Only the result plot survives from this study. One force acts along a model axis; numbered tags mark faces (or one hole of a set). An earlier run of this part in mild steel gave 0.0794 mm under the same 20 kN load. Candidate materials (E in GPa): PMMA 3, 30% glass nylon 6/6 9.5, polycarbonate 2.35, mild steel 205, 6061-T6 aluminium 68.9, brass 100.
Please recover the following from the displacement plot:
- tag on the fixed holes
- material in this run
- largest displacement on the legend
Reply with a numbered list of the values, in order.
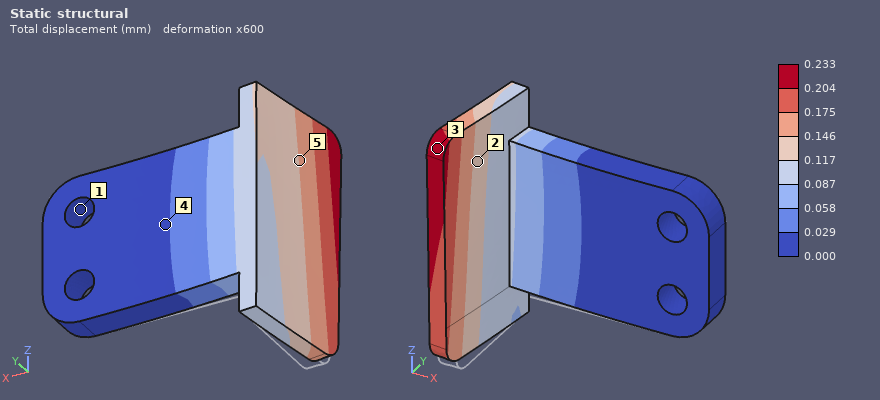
1. 1
2. 6061-T6 aluminium
3. 0.233 mm
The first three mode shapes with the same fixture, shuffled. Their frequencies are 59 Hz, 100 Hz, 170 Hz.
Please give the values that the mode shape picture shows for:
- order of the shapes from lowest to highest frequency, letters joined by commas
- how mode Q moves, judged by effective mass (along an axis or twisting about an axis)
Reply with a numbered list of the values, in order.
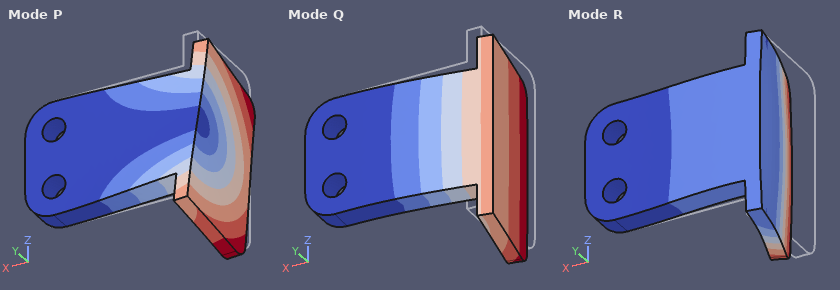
1. Q, P, R
2. along Y
